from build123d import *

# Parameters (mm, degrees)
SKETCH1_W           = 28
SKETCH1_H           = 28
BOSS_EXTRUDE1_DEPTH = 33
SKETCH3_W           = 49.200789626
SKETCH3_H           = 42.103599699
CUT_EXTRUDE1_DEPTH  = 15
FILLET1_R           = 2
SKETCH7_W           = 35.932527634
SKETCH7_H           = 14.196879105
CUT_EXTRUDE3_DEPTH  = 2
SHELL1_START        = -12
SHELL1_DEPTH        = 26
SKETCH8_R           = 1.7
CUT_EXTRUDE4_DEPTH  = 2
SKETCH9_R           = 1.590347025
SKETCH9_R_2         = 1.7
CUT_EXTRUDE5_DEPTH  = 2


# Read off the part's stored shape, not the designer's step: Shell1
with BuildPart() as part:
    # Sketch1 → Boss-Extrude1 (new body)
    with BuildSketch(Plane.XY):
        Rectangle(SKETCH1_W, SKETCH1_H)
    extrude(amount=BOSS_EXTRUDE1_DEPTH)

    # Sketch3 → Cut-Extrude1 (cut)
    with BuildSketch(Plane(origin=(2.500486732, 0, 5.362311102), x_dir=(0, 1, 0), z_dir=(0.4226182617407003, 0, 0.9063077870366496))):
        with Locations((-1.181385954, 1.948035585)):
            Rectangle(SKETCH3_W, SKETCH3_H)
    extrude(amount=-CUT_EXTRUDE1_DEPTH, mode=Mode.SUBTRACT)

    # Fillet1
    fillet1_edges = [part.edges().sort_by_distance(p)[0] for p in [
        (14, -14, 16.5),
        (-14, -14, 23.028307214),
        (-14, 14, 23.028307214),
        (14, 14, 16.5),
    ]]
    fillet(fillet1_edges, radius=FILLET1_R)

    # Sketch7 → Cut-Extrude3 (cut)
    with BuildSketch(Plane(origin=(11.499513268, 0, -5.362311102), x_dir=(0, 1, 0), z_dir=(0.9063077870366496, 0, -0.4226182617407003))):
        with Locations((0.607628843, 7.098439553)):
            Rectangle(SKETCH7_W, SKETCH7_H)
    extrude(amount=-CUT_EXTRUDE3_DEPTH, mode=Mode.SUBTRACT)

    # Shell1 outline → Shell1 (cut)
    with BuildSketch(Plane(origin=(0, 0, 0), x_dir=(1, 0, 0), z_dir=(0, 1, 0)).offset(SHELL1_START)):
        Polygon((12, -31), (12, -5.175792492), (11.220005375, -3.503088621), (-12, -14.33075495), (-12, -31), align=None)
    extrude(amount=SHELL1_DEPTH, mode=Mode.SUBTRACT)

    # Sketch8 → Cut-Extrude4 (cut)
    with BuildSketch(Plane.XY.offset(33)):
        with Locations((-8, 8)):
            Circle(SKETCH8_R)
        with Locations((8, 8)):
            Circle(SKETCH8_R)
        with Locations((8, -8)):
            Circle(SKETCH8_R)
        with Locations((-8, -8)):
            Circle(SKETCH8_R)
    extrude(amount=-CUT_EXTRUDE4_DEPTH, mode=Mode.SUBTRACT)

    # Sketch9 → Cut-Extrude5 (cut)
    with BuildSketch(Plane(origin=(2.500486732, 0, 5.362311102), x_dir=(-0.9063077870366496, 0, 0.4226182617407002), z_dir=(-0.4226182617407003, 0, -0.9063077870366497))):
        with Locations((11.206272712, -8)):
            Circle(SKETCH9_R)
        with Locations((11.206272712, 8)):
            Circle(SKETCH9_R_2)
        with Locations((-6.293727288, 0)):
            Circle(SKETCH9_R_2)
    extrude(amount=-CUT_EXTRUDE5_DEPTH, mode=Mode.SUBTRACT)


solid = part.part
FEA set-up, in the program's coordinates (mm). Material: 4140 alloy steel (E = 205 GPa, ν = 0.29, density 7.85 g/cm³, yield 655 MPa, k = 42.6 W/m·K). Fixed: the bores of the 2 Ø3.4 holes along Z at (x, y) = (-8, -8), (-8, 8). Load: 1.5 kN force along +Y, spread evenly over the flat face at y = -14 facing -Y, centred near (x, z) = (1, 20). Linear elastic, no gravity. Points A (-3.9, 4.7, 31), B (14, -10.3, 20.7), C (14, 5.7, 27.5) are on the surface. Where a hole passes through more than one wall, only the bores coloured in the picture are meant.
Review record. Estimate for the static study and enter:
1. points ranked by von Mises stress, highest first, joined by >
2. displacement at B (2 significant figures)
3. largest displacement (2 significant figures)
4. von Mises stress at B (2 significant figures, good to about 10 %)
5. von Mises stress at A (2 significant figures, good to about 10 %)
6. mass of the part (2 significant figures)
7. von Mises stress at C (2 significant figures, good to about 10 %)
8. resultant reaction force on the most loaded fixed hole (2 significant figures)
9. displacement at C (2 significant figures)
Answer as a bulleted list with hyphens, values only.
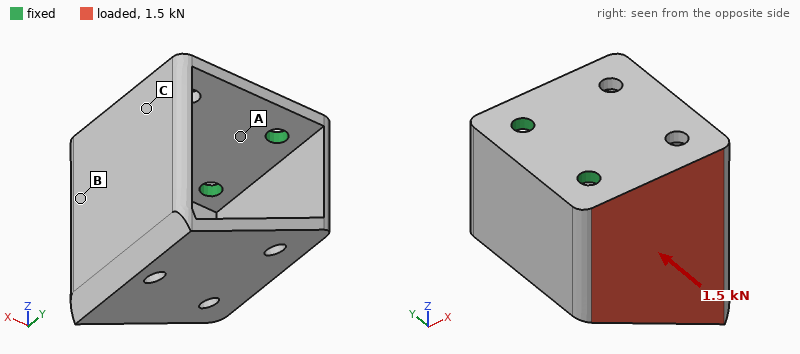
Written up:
- A > C > B
- 0.052 mm
- 0.16 mm
- 35 MPa
- 110 MPa
- 51 g
- 68 MPa
- 1.4 kN
- 0.067 mm
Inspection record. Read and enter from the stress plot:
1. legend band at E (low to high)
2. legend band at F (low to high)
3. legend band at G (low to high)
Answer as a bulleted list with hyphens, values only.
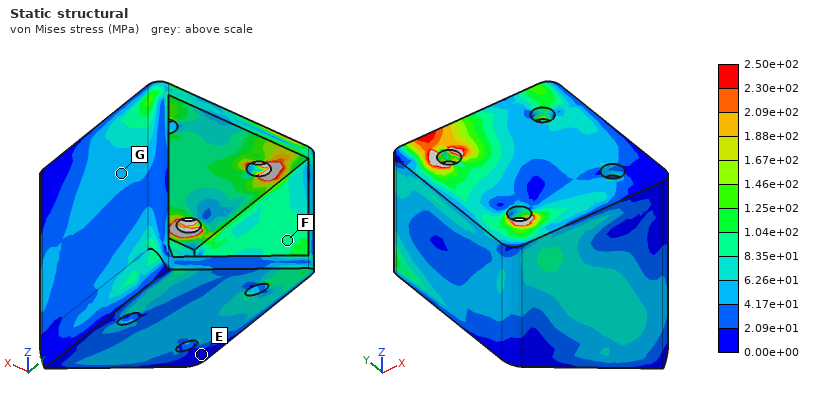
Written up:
- 0.00e+00 to 2.09e+01 MPa
- 8.35e+01 to 1.04e+02 MPa
- 4.17e+01 to 6.26e+01 MPa
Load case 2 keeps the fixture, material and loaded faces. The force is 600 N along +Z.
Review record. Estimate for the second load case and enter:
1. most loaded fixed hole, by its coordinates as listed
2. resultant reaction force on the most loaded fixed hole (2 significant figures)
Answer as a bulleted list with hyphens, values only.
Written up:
- (-8, -8)
- 700 N
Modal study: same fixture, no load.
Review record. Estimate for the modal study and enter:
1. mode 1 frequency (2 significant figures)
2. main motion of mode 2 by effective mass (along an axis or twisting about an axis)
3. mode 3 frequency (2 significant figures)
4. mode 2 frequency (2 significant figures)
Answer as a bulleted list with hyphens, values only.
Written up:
- 1500 Hz
- along Y
- 7000 Hz
- 2400 Hz
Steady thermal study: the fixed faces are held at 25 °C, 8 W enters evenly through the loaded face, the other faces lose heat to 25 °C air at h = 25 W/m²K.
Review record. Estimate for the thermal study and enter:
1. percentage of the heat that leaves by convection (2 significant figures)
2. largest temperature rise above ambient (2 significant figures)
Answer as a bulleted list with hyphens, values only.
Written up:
- 31 %
- 29 K
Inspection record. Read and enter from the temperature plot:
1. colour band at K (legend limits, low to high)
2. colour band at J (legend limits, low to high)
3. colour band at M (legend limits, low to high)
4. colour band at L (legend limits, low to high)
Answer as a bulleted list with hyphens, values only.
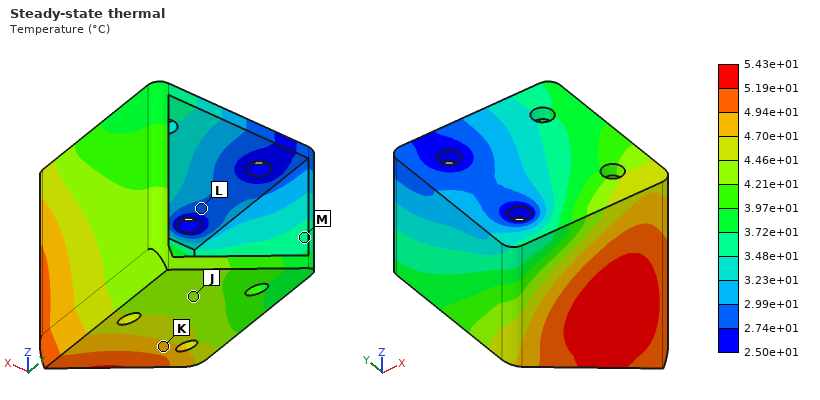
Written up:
- 4.70e+01 to 4.94e+01 °C
- 4.21e+01 to 4.46e+01 °C
- 3.48e+01 to 3.72e+01 °C
- 2.74e+01 to 2.99e+01 °C
